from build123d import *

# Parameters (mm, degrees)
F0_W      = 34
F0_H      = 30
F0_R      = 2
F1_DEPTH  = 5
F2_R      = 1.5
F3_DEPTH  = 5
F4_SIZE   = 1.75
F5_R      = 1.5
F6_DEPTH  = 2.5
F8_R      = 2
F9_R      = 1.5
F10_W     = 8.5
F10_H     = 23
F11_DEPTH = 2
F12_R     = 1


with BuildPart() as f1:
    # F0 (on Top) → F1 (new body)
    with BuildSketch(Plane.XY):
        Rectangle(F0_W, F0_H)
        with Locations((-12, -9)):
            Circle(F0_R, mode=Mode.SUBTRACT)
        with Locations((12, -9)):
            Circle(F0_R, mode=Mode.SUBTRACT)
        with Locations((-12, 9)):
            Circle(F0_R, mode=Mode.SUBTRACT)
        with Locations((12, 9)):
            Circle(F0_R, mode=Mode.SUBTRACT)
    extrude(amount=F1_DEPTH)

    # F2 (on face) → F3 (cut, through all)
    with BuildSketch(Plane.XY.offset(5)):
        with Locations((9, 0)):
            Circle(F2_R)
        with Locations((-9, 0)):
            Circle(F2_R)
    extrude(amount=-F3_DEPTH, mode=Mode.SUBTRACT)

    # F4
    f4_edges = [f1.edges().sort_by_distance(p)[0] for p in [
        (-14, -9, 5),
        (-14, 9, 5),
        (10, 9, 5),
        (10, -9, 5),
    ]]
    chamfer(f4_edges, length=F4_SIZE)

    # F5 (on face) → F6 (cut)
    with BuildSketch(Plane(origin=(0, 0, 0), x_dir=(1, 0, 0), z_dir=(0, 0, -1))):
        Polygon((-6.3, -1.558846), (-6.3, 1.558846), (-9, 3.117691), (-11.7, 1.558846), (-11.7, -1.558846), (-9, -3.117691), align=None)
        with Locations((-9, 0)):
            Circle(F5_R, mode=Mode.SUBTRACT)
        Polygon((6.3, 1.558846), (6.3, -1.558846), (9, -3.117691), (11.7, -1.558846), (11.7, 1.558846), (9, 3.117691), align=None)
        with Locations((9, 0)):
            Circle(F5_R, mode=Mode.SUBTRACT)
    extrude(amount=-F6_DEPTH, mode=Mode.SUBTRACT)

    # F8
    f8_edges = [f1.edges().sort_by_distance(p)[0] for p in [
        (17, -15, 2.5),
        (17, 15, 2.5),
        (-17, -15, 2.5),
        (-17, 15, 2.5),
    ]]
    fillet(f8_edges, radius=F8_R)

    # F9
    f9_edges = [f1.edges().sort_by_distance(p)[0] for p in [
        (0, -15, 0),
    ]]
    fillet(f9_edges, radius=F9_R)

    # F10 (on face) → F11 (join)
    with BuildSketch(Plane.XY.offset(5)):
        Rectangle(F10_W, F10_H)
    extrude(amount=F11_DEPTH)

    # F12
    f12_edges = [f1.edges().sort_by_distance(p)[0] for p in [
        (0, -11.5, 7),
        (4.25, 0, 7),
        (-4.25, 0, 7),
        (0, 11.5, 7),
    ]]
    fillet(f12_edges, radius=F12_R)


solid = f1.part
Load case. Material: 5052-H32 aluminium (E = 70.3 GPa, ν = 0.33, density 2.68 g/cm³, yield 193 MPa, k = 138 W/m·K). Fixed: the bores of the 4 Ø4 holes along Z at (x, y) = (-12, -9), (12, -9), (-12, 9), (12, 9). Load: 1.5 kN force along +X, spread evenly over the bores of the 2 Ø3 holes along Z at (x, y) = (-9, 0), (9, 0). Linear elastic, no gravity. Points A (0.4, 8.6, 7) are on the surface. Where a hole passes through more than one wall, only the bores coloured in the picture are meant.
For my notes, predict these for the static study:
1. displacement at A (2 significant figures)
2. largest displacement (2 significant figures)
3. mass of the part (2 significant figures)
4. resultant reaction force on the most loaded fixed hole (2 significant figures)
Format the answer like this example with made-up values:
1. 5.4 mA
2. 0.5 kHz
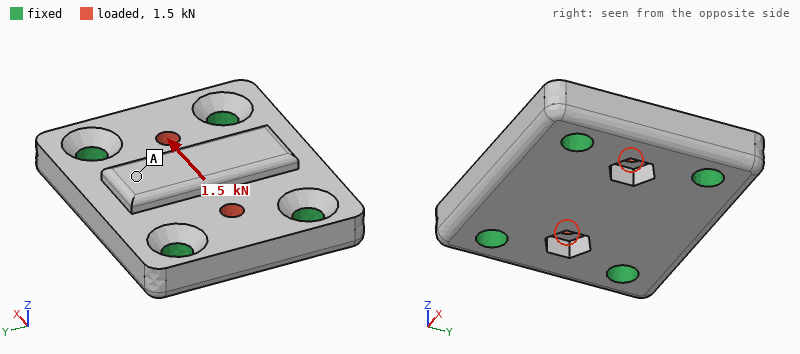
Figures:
1. 0.59 µm
2. 3.3 µm
3. 13 g
4. 390 N
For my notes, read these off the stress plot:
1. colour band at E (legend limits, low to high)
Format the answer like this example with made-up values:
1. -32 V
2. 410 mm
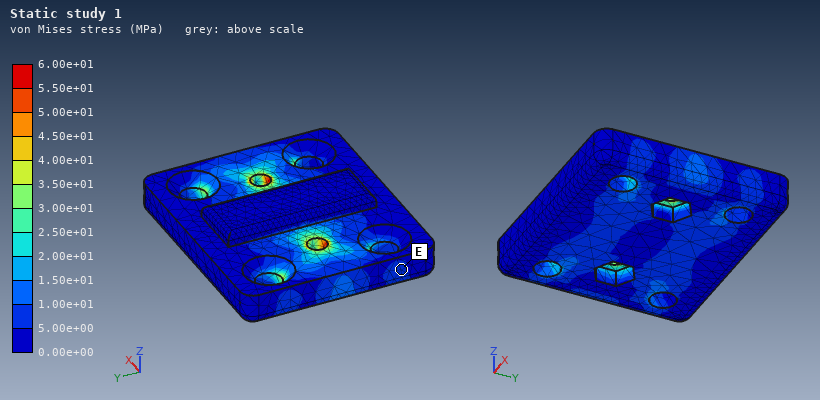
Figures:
1. 5.00e+00 to 1.00e+01 MPa
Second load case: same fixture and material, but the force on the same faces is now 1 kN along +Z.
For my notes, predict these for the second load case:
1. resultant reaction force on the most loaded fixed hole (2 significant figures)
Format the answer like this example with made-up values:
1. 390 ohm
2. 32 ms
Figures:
1. 290 N
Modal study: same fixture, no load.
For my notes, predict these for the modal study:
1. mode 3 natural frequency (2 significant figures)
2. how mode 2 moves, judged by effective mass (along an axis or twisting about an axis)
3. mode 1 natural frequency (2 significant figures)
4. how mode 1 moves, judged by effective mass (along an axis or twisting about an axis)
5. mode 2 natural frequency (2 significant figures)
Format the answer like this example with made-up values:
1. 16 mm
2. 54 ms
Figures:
1. 49 kHz
2. twisting about X
3. 31 kHz
4. along Z
5. 36 kHz
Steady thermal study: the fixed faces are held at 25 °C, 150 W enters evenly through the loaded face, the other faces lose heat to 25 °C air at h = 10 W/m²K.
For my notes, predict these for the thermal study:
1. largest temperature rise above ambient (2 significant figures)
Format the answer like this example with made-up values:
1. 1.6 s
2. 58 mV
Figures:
1. 65 K
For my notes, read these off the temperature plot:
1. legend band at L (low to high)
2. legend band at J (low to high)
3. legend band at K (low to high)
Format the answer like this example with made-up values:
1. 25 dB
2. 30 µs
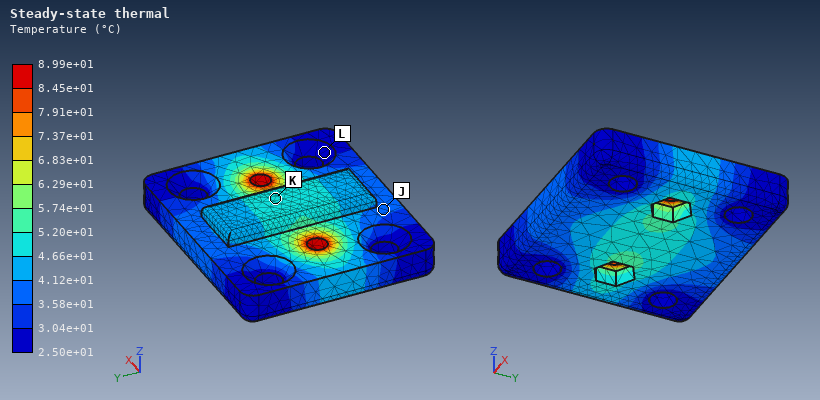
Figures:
1. 2.50e+01 to 3.04e+01 °C
2. 3.58e+01 to 4.12e+01 °C
3. 4.66e+01 to 5.20e+01 °C
